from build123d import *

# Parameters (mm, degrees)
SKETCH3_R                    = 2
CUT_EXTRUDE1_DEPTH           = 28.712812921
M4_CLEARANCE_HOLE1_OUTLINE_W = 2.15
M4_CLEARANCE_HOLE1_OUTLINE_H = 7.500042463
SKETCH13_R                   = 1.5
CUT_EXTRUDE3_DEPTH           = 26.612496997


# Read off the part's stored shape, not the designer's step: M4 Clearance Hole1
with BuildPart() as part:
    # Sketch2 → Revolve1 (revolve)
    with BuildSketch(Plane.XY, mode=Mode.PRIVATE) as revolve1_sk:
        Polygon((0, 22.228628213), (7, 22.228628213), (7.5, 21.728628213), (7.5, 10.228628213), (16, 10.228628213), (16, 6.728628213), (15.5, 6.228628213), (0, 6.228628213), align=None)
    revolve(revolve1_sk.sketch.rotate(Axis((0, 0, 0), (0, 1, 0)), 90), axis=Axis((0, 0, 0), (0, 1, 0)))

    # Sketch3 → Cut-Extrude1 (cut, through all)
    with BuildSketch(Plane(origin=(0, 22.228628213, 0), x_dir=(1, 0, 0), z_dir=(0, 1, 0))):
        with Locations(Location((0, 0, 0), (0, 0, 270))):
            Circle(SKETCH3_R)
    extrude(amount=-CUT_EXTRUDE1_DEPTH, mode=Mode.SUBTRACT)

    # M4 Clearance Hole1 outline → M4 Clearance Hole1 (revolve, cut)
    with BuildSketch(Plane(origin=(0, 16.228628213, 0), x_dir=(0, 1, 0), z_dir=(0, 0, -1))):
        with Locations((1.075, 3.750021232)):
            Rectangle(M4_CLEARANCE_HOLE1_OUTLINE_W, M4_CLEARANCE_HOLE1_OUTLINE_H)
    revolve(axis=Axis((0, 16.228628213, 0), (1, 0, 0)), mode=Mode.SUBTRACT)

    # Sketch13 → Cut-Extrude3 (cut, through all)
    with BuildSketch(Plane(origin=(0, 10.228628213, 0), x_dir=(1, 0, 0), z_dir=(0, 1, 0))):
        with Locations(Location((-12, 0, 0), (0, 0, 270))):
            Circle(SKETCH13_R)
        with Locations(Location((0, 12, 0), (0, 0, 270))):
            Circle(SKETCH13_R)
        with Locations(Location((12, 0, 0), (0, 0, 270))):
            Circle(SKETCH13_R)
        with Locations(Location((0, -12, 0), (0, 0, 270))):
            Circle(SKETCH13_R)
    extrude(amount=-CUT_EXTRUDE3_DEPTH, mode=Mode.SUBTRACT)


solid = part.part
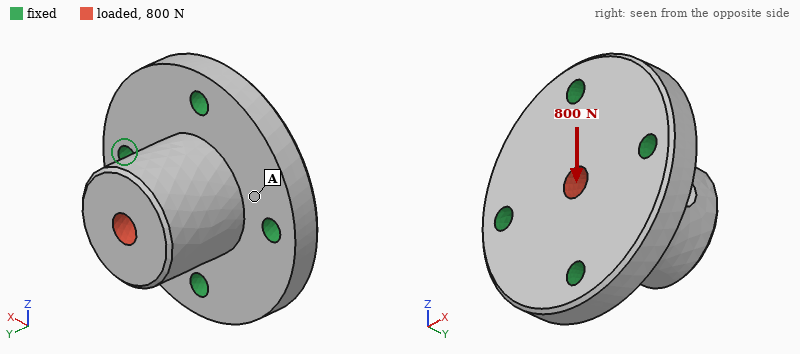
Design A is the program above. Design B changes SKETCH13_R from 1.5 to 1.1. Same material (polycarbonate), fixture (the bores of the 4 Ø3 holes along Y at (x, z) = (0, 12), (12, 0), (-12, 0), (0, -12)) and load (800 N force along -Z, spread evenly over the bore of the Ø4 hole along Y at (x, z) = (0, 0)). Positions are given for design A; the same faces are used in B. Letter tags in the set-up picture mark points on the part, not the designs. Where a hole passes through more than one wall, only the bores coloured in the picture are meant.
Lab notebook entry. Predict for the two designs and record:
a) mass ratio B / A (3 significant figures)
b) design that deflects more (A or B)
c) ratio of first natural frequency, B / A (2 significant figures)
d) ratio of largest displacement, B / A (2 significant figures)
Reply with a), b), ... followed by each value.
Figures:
a) 1.01
b) B
c) 0.95
d) 1.1
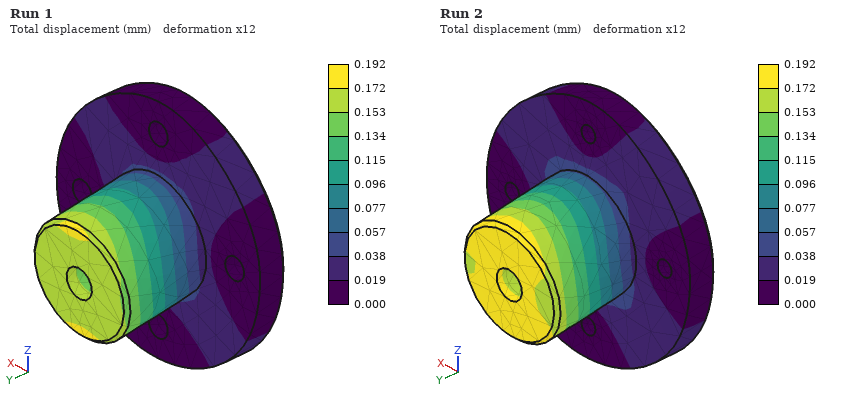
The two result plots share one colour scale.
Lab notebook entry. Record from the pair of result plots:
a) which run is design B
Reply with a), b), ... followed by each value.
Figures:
a) Run 2
